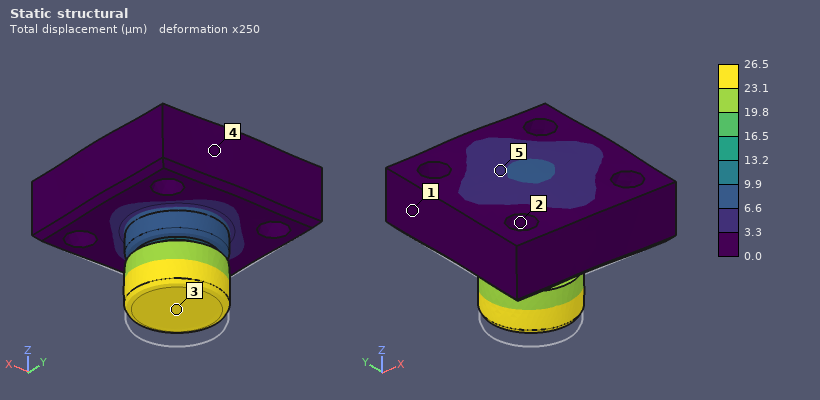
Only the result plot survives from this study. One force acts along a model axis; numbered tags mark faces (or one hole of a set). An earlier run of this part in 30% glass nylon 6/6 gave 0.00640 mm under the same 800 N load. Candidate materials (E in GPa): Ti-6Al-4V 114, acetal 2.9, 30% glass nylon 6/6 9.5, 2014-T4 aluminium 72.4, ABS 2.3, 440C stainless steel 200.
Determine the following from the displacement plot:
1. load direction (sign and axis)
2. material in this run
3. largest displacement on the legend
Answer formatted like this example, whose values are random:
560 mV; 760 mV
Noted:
+Z; ABS; 26.5 µm
